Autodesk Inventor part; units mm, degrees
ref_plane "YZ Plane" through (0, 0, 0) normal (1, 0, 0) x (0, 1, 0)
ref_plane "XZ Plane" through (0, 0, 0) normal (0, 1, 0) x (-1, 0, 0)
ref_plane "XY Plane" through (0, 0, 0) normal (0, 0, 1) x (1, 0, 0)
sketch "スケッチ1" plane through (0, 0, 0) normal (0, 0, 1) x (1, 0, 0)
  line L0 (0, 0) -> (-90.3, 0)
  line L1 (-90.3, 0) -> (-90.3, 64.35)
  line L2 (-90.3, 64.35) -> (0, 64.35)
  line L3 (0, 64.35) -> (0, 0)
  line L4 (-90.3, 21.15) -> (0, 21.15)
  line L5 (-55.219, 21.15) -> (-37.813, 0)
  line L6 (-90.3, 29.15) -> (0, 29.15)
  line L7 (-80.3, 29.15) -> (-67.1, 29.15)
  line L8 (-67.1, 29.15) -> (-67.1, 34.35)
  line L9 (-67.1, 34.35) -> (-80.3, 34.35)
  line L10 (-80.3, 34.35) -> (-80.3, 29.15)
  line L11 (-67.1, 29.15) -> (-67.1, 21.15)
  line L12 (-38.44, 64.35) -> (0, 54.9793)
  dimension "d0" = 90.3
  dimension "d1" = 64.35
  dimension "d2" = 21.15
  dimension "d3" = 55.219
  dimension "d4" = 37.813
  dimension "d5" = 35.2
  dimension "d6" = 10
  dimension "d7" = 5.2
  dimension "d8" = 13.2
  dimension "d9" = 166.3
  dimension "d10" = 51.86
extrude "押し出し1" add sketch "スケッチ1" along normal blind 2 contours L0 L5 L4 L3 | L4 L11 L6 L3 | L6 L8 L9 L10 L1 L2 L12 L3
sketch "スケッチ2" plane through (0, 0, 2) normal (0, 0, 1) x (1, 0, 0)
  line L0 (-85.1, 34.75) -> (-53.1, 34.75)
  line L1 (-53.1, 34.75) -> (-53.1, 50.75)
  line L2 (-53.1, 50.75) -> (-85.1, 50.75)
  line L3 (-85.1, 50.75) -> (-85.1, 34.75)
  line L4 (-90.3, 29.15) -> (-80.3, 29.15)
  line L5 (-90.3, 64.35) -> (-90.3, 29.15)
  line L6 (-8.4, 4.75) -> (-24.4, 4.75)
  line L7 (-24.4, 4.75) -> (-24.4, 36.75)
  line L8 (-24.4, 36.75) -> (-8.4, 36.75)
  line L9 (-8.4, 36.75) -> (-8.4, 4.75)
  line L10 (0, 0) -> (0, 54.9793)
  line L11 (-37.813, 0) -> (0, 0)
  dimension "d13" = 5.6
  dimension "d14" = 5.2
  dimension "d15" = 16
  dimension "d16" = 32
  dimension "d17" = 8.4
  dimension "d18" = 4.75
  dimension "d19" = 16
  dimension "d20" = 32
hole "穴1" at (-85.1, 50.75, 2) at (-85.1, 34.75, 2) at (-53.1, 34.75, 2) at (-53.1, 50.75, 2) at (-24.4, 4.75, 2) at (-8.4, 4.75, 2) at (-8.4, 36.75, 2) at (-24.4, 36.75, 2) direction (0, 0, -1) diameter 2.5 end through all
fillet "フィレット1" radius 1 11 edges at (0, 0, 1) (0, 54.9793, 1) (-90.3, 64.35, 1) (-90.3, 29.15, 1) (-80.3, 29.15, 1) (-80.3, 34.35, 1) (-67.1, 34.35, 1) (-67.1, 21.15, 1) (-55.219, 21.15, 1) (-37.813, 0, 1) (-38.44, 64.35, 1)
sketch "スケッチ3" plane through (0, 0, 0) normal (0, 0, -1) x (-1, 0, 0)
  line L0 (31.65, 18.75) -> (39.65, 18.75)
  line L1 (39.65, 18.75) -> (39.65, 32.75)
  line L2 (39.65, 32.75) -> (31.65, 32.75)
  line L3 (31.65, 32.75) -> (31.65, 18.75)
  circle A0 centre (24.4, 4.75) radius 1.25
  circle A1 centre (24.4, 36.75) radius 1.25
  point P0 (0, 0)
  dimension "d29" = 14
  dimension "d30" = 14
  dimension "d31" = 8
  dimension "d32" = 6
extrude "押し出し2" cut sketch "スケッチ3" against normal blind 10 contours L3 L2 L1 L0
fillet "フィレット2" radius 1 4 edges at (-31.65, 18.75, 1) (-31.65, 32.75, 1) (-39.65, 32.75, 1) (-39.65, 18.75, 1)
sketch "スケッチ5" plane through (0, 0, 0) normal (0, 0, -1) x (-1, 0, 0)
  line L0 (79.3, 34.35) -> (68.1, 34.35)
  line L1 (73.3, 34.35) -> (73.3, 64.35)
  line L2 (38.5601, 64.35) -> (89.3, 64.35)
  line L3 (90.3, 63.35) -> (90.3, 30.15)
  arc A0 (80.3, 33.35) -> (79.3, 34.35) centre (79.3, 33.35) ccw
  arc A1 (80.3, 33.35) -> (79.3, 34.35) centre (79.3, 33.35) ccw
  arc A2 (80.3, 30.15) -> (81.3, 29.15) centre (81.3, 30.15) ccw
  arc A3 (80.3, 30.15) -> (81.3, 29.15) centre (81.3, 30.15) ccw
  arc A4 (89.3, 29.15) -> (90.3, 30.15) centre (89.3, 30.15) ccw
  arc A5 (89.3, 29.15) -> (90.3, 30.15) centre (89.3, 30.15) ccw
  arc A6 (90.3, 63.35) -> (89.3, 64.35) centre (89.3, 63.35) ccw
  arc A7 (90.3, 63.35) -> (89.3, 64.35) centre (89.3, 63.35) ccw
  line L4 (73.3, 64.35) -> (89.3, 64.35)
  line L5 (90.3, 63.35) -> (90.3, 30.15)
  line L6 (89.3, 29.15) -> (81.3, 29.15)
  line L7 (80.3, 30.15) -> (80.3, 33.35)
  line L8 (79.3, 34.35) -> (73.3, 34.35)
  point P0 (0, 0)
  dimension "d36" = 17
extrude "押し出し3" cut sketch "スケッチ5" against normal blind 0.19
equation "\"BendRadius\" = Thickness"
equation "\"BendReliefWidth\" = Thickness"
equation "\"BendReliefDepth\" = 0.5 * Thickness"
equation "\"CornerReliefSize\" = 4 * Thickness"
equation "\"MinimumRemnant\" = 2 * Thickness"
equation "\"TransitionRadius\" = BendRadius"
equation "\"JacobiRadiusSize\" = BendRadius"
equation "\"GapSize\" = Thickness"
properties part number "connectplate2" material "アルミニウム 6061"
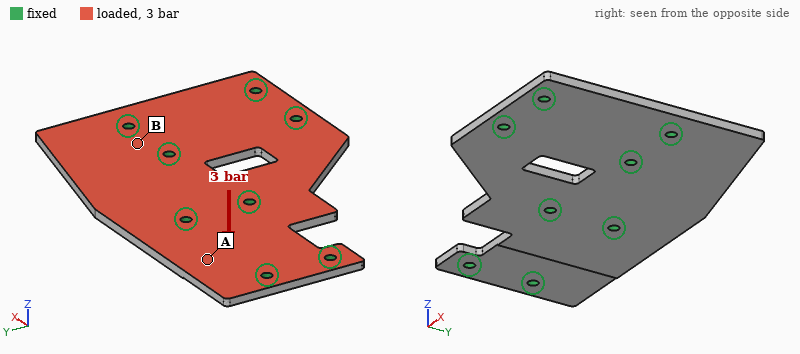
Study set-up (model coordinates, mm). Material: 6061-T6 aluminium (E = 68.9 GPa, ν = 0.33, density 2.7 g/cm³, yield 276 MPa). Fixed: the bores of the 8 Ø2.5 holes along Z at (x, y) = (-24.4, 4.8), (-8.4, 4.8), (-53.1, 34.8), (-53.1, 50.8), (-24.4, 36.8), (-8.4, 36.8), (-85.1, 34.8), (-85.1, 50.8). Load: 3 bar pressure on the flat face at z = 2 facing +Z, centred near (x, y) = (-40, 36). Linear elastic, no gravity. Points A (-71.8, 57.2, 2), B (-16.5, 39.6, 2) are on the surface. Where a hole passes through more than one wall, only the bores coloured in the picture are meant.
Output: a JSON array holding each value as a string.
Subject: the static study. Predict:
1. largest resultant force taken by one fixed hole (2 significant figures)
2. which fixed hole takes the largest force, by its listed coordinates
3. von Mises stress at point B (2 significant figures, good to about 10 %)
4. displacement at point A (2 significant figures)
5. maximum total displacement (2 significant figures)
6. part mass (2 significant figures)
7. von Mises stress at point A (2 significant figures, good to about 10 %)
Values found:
["250 N", "(-53.1, 50.8)", "52 MPa", "0.035 mm", "0.16 mm", "23 g", "20 MPa"]
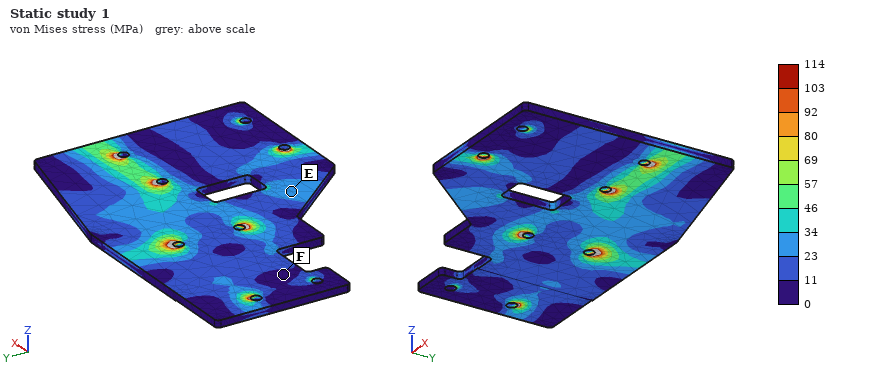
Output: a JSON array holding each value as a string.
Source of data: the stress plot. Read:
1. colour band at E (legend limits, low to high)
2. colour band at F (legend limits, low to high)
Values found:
["23 to 34 MPa", "0 to 11 MPa"]
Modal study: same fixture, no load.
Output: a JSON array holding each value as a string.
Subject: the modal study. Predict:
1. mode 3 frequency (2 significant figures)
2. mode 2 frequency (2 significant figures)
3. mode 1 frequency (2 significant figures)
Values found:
["6300 Hz", "5400 Hz", "3800 Hz"]
